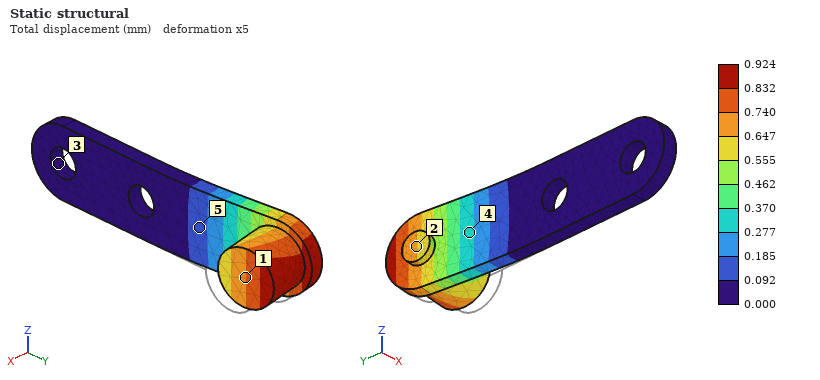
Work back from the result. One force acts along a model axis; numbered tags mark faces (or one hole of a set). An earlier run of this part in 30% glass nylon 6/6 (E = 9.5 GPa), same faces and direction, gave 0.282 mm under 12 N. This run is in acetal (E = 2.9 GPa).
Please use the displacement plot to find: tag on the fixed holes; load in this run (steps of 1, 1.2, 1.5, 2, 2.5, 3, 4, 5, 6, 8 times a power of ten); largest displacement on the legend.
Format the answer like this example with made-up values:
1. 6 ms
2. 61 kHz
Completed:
1. 3
2. 12 N
3. 0.924 mm
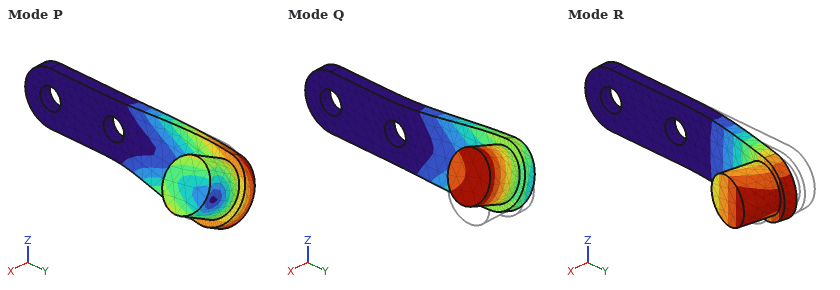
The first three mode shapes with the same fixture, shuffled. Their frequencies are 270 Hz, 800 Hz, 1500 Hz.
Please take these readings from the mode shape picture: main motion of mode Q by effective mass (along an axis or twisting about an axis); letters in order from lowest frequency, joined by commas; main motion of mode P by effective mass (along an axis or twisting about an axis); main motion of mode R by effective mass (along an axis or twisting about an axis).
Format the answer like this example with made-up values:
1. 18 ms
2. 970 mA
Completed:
1. along Z
2. R, Q, P
3. along Z
4. along X
